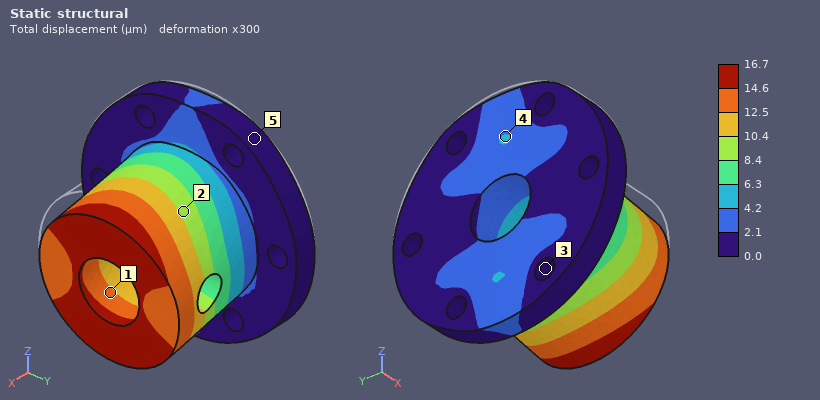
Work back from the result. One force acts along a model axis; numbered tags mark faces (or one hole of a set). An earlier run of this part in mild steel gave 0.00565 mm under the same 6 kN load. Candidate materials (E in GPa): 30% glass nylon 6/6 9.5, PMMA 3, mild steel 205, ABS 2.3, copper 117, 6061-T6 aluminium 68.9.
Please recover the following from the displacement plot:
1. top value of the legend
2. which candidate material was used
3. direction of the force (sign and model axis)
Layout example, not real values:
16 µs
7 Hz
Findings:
16.7 µm
6061-T6 aluminium
-Z
